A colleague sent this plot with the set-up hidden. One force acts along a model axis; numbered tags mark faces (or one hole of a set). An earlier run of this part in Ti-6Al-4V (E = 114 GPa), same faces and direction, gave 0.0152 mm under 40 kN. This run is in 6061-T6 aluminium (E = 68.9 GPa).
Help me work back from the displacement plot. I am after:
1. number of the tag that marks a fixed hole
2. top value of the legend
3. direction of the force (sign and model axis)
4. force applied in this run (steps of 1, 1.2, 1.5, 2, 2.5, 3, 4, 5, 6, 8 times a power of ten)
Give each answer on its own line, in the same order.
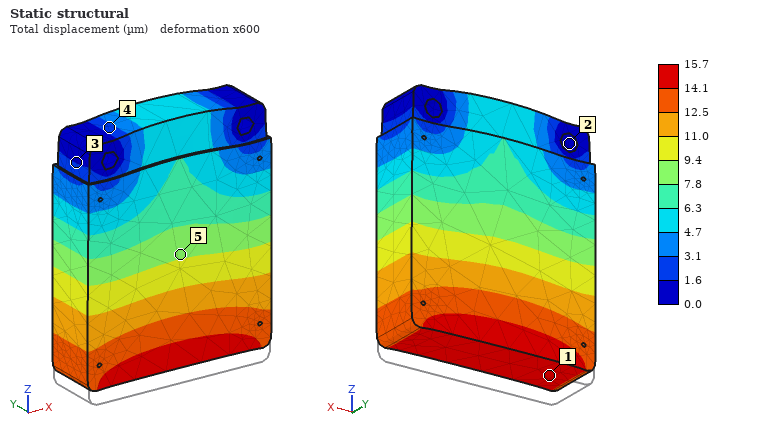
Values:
2
15.7 µm
+Z
25 kN
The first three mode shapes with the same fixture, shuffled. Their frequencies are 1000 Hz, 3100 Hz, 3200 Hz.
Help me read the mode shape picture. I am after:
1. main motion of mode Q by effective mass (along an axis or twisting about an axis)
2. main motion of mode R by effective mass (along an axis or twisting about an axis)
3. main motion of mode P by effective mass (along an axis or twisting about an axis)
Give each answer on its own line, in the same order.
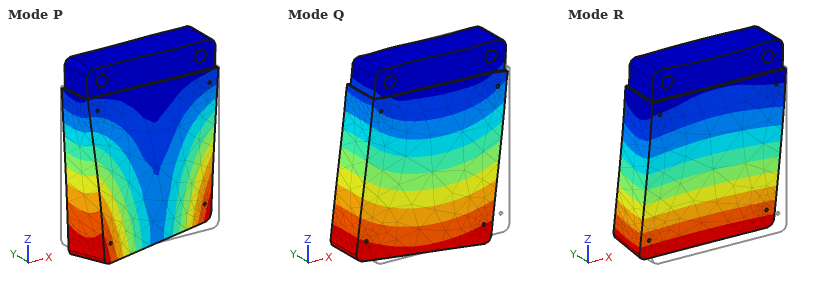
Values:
along X
along Y
twisting about Z
